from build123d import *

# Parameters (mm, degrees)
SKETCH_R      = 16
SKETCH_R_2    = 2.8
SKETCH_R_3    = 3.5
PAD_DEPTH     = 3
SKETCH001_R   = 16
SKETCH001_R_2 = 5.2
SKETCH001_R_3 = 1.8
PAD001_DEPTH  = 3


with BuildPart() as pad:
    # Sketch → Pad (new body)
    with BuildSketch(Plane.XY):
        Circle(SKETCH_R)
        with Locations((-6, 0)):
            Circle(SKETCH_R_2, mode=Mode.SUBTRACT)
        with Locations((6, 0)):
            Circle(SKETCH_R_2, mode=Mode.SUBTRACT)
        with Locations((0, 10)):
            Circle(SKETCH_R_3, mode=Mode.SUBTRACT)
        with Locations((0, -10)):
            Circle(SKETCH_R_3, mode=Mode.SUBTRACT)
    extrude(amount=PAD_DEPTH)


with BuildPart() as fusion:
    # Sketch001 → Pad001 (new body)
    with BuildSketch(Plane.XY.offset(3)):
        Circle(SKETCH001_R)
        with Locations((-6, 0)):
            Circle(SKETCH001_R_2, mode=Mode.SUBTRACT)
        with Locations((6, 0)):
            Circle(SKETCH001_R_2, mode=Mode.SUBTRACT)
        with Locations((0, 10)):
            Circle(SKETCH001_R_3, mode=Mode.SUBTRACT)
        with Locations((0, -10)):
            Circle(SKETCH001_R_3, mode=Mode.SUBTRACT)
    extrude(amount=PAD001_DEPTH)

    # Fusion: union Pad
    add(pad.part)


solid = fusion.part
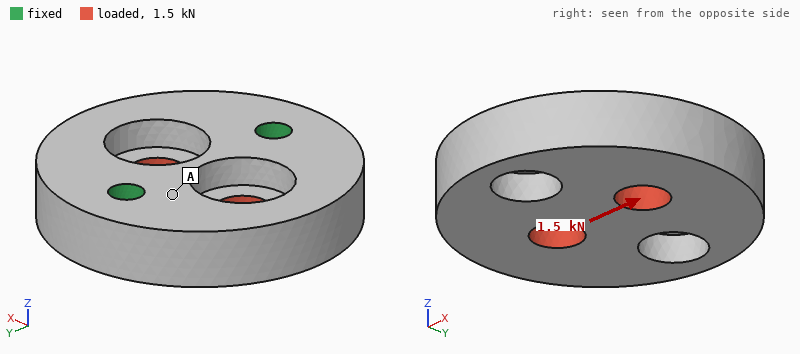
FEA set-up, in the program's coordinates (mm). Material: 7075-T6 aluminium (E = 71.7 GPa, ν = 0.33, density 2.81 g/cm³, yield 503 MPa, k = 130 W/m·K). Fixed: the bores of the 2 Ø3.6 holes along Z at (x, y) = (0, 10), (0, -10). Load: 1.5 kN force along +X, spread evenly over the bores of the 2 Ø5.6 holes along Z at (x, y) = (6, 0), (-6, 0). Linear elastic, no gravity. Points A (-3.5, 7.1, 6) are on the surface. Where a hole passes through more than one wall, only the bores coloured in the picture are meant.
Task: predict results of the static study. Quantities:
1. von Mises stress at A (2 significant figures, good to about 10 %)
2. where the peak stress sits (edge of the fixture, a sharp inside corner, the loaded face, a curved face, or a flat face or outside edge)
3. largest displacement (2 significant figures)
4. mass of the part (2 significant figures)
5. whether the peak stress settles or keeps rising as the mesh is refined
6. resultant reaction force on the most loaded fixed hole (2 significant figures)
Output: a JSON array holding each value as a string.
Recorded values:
["16 MPa", "edge of the fixture", "24 µm", "11 g", "keeps rising", "750 N"]
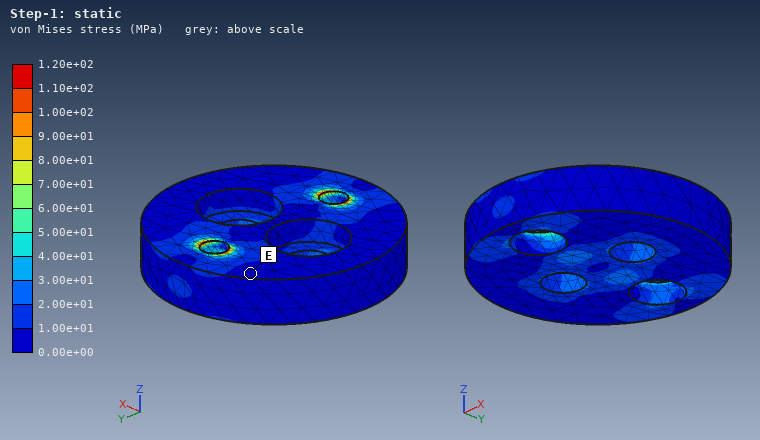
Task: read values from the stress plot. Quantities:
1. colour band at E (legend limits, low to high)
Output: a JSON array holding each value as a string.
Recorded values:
["0.00e+00 to 1.00e+01 MPa"]
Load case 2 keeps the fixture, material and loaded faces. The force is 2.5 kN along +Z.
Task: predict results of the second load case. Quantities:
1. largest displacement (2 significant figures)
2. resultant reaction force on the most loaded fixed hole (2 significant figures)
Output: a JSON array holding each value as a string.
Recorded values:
["26 µm", "1.5 kN"]
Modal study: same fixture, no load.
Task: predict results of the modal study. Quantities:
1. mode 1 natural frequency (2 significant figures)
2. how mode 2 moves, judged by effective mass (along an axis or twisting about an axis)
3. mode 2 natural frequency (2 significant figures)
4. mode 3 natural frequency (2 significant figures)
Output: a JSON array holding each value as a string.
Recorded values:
["10 kHz", "along Z", "17 kHz", "25 kHz"]
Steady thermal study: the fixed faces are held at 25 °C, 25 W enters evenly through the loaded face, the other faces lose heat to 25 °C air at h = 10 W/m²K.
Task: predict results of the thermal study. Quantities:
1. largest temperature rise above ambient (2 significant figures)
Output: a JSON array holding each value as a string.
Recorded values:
["14 K"]
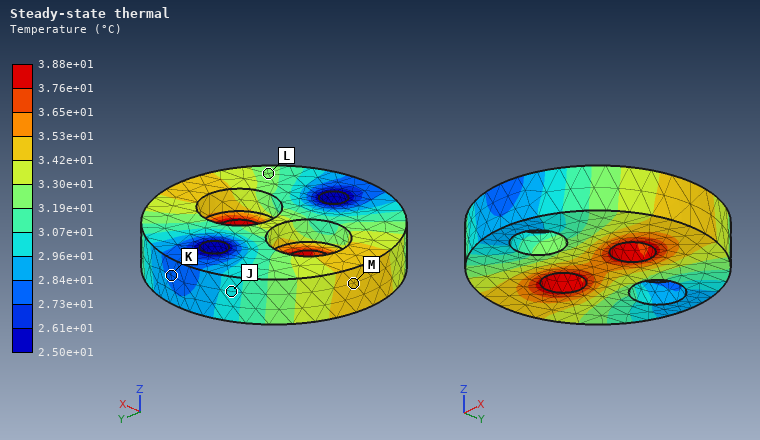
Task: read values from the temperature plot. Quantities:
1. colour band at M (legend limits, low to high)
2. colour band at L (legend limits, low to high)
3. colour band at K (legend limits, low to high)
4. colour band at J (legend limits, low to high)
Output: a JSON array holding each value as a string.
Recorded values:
["3.42e+01 to 3.53e+01 °C", "3.19e+01 to 3.30e+01 °C", "2.73e+01 to 2.84e+01 °C", "2.96e+01 to 3.07e+01 °C"]
